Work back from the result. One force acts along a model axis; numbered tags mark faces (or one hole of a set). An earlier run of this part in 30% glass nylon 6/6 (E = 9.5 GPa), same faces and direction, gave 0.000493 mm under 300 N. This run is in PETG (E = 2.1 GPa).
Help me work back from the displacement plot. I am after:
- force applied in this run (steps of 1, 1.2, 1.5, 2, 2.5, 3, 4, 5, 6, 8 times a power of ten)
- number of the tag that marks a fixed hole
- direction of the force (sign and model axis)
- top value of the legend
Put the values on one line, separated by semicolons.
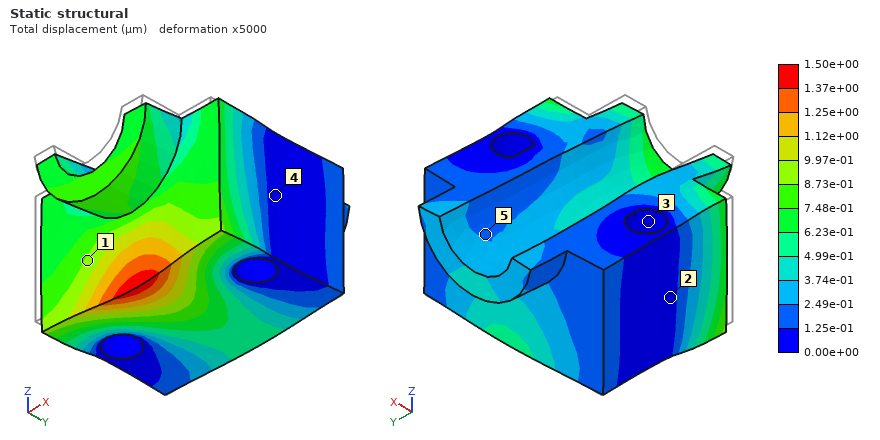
200 N; 3; +Y; 1.50e+00 µm
